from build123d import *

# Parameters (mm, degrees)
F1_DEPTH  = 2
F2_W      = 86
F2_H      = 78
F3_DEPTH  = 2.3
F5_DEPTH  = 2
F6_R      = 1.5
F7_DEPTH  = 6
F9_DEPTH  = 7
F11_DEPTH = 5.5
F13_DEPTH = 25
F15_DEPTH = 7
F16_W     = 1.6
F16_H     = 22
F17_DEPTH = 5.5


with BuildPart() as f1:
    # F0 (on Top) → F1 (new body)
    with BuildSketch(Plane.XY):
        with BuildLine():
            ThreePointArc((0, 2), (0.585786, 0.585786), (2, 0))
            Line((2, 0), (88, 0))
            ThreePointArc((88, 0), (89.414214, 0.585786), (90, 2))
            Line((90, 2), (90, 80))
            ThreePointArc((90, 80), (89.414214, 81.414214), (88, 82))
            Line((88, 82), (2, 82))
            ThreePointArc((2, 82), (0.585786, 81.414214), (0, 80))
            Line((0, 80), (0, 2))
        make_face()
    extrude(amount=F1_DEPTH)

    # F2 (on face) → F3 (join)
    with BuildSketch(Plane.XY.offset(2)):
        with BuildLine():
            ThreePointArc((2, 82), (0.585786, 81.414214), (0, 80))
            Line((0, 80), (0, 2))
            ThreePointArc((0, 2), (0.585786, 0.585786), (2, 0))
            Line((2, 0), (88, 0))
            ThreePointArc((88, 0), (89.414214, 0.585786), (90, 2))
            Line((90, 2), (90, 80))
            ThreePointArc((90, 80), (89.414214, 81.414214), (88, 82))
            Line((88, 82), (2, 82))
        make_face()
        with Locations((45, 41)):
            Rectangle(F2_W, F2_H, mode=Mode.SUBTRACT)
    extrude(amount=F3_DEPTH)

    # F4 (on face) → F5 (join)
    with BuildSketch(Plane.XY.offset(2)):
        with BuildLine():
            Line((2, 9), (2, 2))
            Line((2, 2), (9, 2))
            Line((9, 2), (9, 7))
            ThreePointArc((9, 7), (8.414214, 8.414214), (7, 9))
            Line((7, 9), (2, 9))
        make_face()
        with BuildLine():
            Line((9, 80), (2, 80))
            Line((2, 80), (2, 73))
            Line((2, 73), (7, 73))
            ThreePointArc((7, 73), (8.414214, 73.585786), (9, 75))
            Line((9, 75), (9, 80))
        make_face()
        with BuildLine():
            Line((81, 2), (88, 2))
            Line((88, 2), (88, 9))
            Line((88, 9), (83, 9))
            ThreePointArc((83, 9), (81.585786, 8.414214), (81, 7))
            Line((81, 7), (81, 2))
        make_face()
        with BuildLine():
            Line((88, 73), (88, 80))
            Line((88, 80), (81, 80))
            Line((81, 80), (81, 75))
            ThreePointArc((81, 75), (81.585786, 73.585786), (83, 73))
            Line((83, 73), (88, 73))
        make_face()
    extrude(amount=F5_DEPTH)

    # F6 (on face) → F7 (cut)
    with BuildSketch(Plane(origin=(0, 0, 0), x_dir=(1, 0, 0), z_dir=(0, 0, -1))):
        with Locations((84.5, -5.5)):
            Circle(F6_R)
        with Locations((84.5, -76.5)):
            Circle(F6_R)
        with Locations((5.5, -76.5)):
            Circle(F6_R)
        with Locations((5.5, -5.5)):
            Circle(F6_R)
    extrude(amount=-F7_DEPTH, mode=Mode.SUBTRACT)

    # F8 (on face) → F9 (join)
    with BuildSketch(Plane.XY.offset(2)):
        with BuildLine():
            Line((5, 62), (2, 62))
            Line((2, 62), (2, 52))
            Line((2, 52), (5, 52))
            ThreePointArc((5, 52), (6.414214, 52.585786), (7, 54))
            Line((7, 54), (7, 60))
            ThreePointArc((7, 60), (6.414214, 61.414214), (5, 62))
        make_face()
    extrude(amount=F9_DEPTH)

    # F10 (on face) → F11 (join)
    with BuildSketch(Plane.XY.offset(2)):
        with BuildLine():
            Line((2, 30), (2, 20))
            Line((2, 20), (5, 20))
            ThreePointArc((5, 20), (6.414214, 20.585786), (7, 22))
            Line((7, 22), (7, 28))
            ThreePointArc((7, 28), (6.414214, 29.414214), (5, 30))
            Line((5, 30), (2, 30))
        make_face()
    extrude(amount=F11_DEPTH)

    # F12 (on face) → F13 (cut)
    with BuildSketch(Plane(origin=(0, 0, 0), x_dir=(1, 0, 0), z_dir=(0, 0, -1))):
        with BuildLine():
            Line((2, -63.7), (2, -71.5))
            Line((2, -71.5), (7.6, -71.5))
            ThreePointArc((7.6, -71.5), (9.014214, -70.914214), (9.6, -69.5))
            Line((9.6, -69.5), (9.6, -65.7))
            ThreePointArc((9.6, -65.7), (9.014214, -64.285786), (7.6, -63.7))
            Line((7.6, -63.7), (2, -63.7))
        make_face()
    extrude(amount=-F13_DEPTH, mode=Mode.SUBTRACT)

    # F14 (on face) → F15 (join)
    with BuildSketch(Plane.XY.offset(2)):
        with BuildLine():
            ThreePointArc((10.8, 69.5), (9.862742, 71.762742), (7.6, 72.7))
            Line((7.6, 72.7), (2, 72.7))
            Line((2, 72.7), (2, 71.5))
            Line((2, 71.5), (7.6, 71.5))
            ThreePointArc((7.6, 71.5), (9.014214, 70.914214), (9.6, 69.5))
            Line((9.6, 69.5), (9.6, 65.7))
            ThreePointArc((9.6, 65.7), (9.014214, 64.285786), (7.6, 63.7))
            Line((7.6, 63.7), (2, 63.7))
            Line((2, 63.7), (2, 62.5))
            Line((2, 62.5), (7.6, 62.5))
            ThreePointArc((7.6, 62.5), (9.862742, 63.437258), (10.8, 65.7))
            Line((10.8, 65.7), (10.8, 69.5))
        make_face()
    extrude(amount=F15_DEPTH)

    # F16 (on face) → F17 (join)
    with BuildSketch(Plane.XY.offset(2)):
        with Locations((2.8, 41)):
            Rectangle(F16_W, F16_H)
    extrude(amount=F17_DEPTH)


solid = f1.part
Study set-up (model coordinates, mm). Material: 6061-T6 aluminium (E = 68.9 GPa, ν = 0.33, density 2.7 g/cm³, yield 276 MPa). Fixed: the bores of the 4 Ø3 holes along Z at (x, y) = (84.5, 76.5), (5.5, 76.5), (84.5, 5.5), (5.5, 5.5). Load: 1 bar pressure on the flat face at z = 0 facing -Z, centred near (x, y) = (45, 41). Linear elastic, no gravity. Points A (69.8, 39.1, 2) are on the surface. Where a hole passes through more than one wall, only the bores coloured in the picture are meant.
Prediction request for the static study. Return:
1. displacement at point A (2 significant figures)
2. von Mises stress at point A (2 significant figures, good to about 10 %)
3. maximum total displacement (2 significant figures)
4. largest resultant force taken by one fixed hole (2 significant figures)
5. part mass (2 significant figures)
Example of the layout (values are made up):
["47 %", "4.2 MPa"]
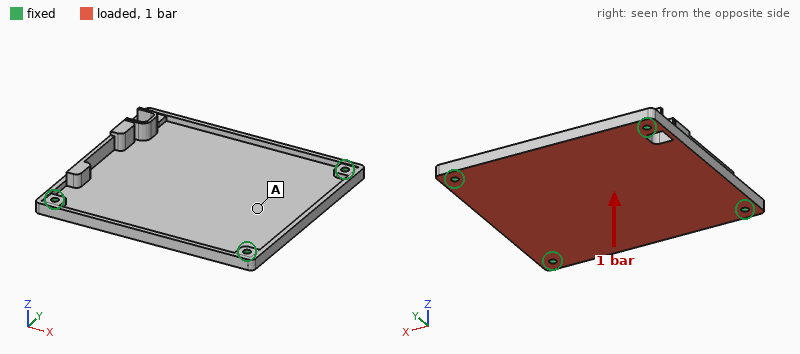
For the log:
["0.22 mm", "28 MPa", "0.32 mm", "230 N", "47 g"]
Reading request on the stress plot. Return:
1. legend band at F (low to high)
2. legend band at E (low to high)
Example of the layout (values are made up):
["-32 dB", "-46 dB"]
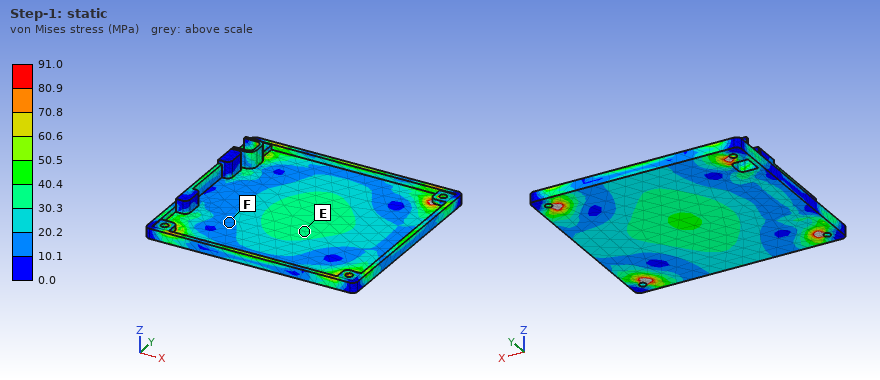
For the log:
["10.1 to 20.2 MPa", "30.3 to 40.4 MPa"]
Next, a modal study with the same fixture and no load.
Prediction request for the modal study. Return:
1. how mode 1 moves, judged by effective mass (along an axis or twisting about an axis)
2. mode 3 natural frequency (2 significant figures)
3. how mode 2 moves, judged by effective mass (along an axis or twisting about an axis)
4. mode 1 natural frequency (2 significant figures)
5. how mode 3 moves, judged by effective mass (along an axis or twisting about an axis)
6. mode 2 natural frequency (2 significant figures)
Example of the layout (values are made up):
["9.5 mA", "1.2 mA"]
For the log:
["along Z", "3000 Hz", "twisting about X", "1500 Hz", "twisting about Y", "2700 Hz"]
